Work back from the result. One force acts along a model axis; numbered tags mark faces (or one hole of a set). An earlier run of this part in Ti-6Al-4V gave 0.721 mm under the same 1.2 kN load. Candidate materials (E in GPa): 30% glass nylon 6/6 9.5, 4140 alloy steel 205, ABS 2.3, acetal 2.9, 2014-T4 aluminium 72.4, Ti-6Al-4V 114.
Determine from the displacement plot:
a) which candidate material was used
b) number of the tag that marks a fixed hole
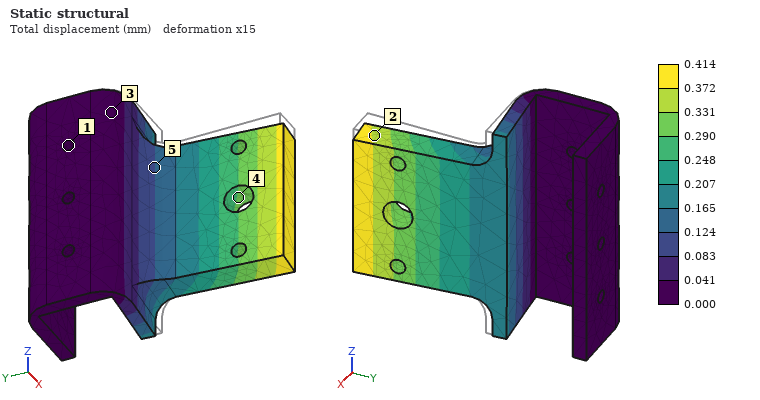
4140 alloy steel
1
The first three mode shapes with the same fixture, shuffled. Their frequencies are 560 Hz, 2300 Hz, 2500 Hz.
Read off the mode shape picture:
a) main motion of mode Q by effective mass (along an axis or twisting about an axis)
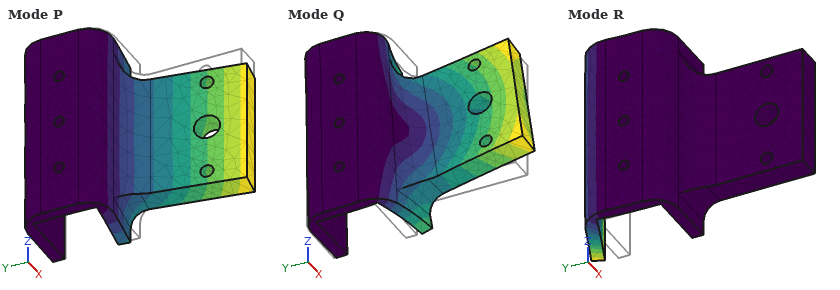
along Z
